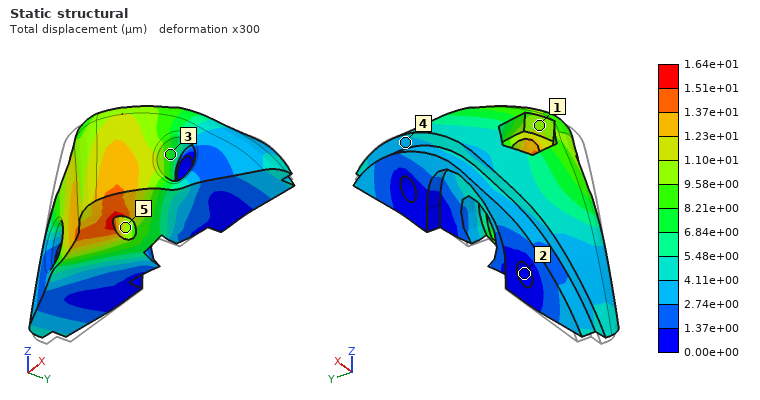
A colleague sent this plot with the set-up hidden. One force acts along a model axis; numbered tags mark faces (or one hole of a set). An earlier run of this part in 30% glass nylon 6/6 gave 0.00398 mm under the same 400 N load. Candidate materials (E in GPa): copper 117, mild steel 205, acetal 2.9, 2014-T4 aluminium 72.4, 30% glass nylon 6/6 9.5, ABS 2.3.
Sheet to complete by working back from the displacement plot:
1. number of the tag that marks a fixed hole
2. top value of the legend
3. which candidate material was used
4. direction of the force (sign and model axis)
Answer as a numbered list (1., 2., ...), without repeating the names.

1. 2
2. 1.64e+01 µm
3. ABS
4. +X
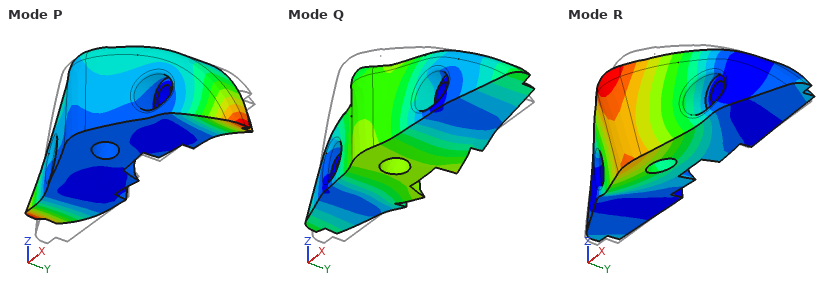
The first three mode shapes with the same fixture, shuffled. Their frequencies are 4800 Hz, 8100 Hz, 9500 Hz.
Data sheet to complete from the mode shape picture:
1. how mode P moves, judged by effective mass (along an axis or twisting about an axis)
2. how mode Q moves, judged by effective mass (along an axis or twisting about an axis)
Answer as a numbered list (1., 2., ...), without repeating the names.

1. along X
2. along Y
